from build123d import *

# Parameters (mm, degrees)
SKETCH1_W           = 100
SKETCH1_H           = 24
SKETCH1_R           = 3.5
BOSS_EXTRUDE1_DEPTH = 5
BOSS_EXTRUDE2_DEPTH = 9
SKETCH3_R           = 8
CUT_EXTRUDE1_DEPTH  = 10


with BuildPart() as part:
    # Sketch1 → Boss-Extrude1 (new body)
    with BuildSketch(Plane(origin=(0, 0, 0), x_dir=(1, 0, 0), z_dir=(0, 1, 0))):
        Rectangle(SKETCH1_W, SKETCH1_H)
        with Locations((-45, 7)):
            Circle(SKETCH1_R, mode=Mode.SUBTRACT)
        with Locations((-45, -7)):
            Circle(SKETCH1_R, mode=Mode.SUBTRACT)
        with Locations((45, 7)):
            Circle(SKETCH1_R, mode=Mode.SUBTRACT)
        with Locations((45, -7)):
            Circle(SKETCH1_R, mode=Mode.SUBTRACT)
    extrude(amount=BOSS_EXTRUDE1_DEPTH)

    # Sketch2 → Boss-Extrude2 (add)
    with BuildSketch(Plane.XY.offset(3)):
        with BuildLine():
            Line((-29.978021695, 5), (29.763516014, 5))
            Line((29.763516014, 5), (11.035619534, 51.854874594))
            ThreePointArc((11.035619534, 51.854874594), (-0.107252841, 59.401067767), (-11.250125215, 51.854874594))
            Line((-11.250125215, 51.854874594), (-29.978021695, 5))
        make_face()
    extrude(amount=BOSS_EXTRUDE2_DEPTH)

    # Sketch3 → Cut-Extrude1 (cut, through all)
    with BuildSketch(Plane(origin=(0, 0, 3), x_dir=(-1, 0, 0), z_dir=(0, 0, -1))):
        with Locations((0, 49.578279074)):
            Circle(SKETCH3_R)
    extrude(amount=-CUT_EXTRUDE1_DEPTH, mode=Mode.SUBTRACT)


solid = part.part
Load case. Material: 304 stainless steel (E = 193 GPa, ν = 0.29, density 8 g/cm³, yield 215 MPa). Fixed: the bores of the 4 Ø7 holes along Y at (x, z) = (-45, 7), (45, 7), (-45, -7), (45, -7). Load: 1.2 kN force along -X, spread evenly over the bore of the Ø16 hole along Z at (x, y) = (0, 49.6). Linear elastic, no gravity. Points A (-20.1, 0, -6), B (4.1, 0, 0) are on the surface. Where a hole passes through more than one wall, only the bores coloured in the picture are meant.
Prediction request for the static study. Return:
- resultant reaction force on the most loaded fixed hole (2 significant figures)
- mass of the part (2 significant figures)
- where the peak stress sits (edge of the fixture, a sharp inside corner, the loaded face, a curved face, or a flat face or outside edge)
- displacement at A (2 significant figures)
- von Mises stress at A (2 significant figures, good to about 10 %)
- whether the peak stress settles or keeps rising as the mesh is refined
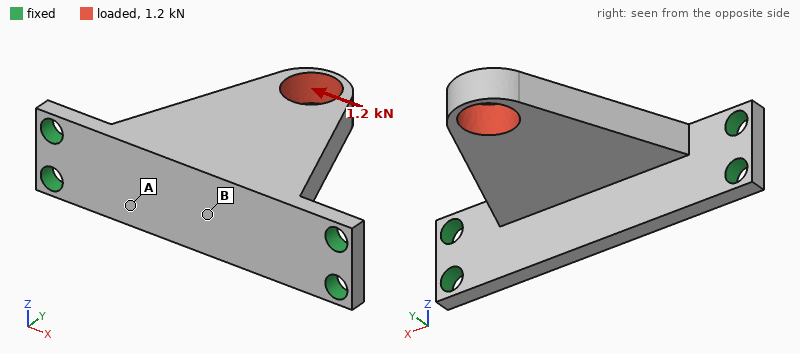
780 N
220 g
edge of the fixture
4.7 µm
15 MPa
keeps rising
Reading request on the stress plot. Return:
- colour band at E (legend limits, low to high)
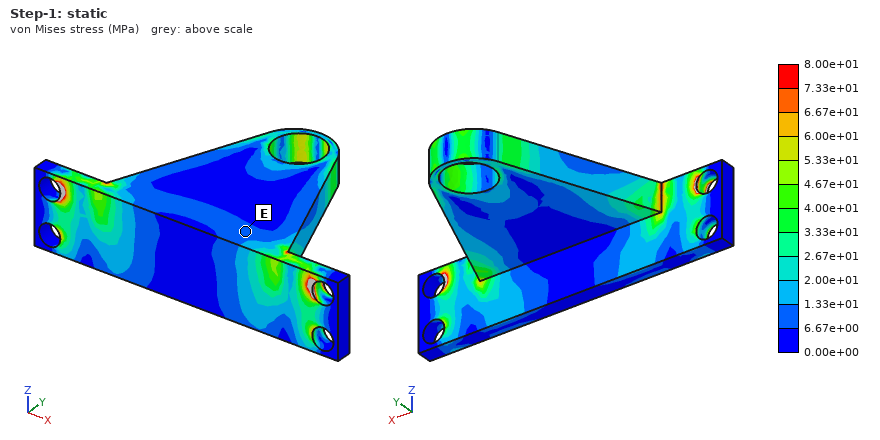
6.67e+00 to 1.33e+01 MPa
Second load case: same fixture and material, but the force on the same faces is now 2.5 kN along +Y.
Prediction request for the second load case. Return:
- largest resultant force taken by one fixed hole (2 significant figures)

1.4 kN
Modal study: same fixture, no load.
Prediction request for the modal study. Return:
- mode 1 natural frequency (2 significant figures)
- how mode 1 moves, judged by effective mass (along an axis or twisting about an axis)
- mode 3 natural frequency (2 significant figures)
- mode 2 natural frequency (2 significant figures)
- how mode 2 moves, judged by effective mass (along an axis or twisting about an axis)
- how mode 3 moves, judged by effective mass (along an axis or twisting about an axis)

1500 Hz
along Z
5600 Hz
4200 Hz
along Y
along X
